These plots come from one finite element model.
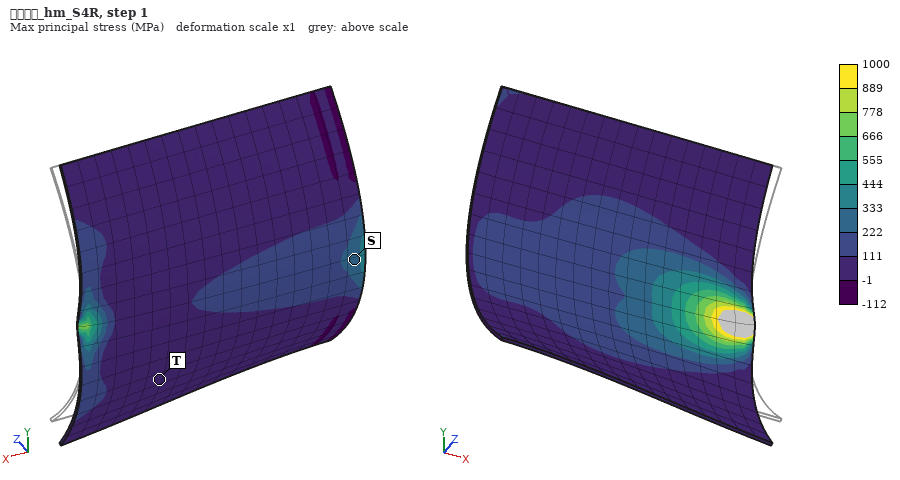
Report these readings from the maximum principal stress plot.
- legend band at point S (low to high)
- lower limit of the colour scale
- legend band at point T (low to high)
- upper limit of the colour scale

222 to 333 MPa
-112 MPa
-1 to 111 MPa
1000 MPa
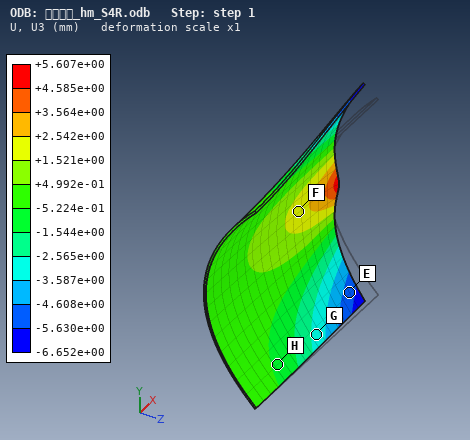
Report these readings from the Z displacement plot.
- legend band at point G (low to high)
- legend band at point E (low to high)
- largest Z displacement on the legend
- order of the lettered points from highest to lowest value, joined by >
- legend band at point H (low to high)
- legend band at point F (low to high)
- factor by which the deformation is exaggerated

-3.587e+00 to -2.565e+00 mm
-5.630e+00 to -4.608e+00 mm
+5.607e+00 mm
F > H > G > E
-1.544e+00 to -5.224e-01 mm
+1.521e+00 to +2.542e+00 mm
1
